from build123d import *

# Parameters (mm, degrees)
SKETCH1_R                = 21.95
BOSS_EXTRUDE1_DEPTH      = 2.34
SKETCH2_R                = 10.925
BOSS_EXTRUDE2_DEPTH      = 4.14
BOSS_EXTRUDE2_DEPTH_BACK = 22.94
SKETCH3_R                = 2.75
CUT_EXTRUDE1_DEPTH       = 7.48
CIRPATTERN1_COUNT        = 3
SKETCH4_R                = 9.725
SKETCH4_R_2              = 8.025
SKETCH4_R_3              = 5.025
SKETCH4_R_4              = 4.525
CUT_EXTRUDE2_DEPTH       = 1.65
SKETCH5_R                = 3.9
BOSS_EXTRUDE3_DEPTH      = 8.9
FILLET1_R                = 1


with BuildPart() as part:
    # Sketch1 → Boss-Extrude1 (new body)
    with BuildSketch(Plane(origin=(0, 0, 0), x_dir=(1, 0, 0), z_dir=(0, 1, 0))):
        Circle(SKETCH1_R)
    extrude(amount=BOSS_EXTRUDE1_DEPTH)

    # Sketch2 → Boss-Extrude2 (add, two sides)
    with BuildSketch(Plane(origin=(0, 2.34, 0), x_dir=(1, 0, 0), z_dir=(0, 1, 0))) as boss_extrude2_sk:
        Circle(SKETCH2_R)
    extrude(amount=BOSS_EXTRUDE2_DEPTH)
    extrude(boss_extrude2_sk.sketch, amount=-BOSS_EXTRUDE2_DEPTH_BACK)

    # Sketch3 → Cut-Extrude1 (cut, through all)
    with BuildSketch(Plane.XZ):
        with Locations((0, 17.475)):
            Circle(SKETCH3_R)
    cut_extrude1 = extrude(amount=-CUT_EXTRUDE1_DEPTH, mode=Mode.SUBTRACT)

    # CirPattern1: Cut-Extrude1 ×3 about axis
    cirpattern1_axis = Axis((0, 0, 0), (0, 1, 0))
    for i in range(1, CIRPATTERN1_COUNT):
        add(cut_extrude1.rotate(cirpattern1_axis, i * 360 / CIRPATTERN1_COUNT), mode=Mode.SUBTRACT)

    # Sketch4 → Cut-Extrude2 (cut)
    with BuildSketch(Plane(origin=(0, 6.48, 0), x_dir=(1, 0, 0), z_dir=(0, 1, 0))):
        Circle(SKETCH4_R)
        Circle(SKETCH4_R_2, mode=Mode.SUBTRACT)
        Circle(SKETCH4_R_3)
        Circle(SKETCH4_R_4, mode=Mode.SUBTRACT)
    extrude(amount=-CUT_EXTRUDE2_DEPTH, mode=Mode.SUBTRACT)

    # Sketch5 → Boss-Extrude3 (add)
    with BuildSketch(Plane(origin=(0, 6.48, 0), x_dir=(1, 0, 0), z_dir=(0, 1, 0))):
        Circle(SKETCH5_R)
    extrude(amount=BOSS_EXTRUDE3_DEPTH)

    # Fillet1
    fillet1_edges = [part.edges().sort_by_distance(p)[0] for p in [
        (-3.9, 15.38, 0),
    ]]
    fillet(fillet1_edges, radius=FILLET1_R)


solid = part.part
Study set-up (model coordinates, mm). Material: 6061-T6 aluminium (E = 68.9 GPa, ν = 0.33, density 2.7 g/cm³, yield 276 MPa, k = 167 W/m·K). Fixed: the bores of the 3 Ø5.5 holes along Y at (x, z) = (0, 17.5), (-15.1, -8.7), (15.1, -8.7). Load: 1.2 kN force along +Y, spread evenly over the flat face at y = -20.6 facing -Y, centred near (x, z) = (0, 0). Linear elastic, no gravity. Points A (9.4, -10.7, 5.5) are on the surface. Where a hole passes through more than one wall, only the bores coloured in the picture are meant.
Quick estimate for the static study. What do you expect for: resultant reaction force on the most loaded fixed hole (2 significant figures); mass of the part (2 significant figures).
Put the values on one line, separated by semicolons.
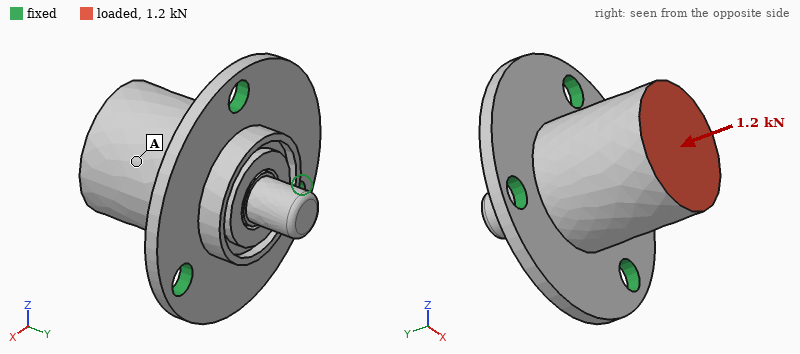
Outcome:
400 N; 35 g
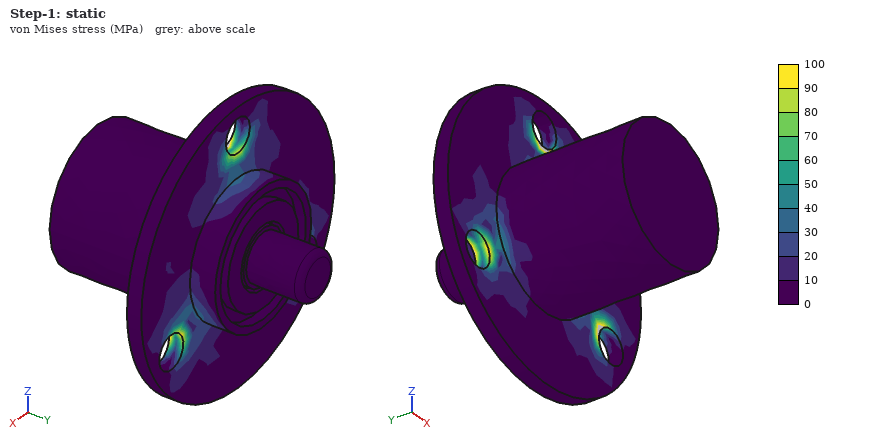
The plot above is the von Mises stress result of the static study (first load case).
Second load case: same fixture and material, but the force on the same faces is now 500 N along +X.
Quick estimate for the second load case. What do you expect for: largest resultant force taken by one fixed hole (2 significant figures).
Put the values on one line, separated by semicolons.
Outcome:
470 N
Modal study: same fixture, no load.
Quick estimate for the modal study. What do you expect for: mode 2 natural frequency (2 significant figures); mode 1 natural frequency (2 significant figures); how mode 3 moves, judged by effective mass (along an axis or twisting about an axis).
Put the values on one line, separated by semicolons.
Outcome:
7600 Hz; 7600 Hz; along Y
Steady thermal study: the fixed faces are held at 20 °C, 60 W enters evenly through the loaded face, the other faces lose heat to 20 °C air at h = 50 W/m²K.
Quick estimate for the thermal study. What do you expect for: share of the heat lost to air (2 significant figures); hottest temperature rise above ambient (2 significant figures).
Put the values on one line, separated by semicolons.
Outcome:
7.2 %; 39 K
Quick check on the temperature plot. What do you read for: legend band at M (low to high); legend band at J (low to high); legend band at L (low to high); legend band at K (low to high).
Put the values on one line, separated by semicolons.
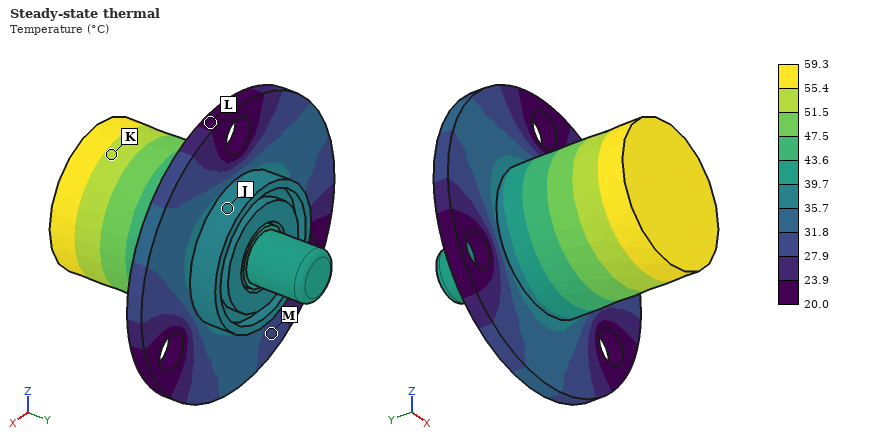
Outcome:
27.9 to 31.8 °C; 35.7 to 39.7 °C; 20.0 to 23.9 °C; 51.5 to 55.4 °C
